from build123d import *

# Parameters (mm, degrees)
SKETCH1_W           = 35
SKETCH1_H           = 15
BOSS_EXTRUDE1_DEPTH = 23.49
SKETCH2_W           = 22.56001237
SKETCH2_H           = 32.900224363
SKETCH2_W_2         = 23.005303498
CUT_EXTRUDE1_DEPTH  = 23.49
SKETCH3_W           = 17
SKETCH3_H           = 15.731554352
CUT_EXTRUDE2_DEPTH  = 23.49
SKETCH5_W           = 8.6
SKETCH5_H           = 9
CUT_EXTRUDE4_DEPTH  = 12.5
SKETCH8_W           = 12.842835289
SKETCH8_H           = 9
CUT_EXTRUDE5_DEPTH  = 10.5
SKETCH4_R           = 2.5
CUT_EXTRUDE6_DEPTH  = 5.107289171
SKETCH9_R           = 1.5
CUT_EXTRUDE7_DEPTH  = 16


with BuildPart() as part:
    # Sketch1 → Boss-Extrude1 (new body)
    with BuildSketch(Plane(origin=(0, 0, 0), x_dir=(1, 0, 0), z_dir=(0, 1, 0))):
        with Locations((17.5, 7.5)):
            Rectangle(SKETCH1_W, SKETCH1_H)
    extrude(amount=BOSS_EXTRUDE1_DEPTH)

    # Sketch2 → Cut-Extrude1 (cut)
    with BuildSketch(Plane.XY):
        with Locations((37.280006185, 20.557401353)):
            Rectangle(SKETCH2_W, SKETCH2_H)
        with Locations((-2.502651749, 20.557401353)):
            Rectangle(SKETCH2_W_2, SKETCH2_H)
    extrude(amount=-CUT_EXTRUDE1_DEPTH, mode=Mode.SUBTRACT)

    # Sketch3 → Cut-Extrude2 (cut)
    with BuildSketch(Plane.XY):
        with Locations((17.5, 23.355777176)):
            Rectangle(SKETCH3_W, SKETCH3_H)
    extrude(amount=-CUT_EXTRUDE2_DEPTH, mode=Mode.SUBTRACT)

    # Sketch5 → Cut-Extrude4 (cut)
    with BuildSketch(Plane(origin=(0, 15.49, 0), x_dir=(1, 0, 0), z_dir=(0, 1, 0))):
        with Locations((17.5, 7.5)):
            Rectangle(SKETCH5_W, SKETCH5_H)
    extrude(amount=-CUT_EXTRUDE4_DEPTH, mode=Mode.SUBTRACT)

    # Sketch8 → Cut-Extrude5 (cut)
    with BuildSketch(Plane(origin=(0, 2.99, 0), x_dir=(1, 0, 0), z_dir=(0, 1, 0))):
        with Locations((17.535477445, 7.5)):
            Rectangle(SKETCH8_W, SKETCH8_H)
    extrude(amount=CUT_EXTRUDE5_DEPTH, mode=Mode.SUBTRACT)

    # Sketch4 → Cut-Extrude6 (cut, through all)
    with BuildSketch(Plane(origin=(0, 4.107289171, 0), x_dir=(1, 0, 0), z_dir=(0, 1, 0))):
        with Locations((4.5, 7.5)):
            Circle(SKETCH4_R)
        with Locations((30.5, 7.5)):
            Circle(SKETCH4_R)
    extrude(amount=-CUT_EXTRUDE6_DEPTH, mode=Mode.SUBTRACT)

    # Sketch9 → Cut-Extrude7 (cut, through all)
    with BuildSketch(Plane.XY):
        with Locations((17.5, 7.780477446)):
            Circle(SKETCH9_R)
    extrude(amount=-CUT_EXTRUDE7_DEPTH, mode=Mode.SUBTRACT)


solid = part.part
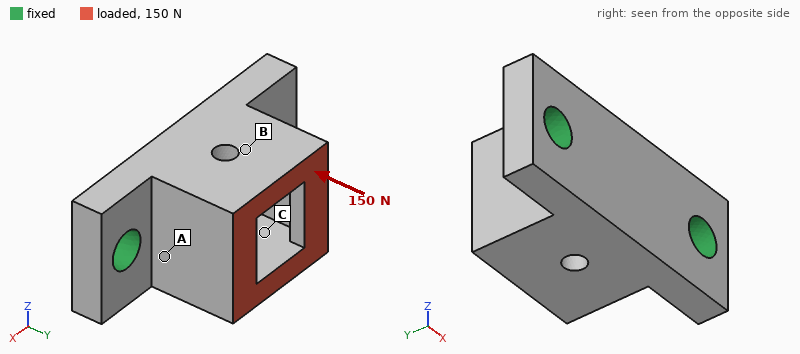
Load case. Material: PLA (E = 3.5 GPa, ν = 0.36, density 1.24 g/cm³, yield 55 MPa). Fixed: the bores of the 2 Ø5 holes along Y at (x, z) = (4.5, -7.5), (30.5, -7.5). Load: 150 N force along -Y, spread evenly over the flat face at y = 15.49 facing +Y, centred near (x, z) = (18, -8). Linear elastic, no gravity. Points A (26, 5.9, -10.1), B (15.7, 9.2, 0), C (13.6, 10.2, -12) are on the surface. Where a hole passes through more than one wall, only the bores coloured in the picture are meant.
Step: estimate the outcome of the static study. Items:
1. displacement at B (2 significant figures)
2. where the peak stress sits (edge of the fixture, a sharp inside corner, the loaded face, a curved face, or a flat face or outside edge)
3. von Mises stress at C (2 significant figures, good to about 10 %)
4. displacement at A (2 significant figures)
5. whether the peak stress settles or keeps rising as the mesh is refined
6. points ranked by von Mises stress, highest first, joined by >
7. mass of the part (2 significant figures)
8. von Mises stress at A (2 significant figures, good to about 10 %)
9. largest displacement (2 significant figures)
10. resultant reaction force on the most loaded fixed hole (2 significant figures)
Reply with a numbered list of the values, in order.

1. 14 µm
2. edge of the fixture
3. 1.3 MPa
4. 10 µm
5. keeps rising
6. A > C > B
7. 4.3 g
8. 3.6 MPa
9. 21 µm
10. 76 N
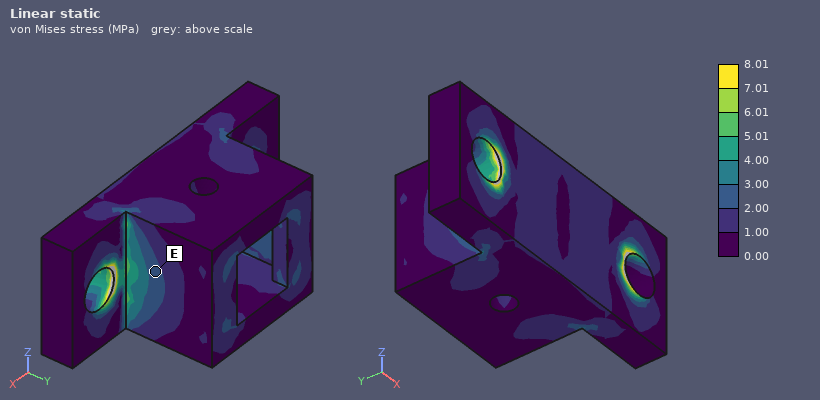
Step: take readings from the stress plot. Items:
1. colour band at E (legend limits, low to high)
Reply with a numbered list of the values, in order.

1. 2.00 to 3.00 MPa
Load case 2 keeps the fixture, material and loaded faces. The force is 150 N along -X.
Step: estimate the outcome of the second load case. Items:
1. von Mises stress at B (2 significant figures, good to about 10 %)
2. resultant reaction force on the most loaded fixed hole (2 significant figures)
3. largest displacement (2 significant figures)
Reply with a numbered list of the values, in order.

1. 3.3 MPa
2. 130 N
3. 57 µm
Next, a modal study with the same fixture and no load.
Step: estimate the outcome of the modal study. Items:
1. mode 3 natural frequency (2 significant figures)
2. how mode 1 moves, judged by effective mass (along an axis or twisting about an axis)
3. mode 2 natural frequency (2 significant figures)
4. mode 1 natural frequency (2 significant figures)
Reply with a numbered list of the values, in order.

1. 9600 Hz
2. along Z
3. 9400 Hz
4. 4500 Hz
